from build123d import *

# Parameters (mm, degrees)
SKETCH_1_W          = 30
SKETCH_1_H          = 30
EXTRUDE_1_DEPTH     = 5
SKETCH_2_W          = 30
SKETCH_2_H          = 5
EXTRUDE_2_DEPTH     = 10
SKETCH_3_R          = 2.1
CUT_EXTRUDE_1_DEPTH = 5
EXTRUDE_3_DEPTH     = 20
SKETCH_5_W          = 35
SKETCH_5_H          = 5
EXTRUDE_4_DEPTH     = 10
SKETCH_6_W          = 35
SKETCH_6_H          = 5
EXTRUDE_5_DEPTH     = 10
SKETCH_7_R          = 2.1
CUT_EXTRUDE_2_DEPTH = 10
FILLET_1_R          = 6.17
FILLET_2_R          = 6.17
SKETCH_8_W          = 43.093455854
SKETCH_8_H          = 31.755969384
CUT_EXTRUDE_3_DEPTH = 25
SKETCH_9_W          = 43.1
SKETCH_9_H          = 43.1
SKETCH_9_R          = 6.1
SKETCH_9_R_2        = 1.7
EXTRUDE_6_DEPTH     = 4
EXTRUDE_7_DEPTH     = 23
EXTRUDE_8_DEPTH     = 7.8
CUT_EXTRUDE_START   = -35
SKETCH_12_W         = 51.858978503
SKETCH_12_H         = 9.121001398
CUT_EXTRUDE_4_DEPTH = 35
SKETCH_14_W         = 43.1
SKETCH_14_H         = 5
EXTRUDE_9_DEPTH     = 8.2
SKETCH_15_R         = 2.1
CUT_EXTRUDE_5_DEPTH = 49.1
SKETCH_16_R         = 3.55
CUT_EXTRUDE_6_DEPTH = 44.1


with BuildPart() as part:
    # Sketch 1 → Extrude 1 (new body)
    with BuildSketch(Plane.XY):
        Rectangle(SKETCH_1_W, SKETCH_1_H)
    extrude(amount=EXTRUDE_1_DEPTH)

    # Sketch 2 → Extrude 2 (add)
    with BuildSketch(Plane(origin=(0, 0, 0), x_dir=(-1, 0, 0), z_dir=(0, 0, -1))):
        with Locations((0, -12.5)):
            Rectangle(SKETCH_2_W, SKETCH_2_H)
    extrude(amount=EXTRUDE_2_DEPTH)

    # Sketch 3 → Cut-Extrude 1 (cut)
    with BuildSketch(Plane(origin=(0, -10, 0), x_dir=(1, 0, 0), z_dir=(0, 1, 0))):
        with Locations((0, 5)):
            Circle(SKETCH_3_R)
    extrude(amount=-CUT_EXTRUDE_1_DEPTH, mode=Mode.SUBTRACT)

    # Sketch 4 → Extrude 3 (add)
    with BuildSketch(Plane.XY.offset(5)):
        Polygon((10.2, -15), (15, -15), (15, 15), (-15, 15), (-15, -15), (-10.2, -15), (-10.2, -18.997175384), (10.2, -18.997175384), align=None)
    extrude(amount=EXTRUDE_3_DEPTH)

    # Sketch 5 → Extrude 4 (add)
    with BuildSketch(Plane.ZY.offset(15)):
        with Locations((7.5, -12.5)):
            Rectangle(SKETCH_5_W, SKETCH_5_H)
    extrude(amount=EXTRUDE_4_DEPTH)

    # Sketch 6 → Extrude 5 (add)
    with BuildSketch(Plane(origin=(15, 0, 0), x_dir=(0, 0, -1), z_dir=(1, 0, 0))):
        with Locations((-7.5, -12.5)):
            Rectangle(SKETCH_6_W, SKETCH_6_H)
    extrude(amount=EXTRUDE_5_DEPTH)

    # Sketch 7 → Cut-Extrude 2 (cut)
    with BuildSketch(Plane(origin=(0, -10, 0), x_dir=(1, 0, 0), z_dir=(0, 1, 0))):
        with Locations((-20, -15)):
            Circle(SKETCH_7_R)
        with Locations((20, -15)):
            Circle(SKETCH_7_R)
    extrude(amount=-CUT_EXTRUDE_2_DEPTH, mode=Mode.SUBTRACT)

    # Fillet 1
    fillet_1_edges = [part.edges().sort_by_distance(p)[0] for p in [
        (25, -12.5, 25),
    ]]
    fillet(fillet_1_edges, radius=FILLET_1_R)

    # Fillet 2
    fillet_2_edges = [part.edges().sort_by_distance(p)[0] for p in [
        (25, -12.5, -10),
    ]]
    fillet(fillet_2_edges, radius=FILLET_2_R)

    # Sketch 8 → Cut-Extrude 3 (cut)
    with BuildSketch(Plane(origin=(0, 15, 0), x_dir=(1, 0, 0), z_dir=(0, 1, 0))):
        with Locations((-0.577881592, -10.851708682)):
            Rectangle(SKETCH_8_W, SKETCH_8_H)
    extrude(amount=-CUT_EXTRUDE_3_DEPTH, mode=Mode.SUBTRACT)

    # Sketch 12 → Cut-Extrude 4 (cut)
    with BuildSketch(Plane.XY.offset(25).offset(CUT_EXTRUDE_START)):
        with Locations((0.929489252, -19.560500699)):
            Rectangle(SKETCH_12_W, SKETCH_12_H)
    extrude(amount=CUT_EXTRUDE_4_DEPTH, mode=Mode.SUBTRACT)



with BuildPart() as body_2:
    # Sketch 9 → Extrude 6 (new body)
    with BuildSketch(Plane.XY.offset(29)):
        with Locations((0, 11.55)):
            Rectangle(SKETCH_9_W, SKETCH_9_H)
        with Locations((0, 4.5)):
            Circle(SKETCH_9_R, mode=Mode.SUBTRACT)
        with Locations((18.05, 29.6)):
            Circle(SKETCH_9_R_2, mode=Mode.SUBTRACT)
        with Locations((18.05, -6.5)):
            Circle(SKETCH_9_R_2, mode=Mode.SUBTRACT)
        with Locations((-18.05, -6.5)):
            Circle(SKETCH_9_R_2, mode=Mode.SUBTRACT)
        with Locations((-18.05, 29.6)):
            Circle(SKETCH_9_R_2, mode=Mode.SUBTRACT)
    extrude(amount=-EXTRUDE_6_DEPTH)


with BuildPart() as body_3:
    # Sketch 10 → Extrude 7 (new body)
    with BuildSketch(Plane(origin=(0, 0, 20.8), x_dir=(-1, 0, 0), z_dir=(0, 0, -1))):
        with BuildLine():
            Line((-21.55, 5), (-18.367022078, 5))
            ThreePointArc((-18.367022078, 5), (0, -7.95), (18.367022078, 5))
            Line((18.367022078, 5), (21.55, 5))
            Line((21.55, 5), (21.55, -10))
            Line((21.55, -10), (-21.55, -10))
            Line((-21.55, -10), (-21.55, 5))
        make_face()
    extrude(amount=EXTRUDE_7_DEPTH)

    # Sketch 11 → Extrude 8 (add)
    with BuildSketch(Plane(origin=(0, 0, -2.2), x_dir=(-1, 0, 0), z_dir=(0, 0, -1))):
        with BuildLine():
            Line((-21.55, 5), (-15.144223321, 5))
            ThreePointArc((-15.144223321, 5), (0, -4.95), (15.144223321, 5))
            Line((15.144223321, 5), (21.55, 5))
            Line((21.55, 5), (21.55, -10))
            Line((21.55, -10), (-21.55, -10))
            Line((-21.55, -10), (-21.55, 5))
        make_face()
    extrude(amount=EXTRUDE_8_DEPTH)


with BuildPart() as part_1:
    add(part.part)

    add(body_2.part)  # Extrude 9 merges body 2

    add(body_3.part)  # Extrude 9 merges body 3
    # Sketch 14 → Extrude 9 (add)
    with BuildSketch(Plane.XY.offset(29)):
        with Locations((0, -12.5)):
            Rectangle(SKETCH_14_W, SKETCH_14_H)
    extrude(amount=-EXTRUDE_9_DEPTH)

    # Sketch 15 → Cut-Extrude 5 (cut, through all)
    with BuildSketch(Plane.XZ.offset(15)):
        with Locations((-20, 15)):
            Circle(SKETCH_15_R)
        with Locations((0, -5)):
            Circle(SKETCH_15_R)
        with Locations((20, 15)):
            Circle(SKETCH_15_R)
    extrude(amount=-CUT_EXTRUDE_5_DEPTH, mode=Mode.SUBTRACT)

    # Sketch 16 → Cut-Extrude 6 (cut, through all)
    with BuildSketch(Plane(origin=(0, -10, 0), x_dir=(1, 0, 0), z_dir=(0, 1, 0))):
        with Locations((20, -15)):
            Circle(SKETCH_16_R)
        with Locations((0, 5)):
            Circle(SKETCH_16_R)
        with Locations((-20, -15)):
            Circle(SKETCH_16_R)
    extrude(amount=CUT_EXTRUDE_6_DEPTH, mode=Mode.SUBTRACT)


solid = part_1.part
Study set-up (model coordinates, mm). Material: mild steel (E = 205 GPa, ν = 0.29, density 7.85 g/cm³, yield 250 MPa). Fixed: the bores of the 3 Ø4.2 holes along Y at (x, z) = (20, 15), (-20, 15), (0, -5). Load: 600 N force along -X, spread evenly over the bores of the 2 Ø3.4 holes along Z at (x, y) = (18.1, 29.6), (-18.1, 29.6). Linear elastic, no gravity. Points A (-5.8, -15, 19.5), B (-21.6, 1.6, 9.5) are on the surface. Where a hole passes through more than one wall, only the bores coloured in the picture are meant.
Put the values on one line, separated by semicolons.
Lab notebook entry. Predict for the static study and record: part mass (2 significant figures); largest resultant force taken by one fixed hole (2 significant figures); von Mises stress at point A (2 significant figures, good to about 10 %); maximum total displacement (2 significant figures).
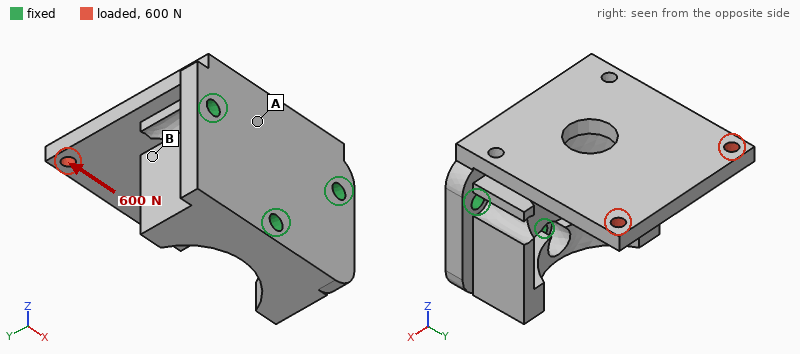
200 g; 770 N; 16 MPa; 27 µm
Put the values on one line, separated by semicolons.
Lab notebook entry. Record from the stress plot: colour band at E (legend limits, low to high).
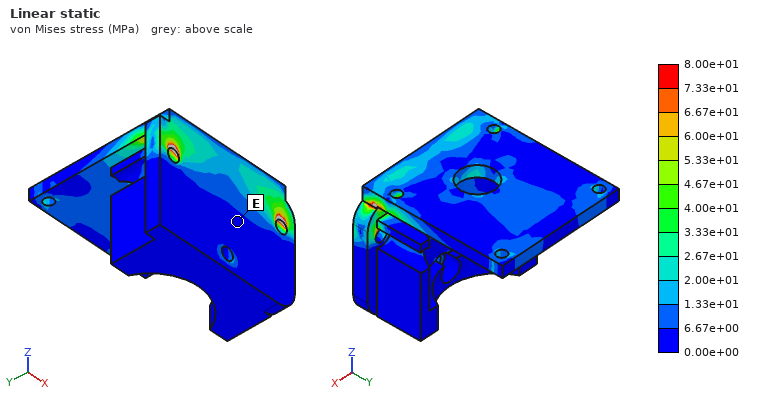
0.00e+00 to 6.67e+00 MPa
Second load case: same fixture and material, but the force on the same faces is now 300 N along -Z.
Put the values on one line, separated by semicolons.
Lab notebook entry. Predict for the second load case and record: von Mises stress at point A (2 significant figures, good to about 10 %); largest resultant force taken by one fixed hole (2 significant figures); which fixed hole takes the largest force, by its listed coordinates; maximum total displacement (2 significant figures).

39 MPa; 450 N; (0, -5); 0.25 mm
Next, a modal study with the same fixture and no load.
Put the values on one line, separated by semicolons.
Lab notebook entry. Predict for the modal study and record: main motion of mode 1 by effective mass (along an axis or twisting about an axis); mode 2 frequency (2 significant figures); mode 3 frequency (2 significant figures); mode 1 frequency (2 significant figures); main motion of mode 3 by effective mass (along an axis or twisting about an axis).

along Z; 3600 Hz; 5500 Hz; 1300 Hz; along X
